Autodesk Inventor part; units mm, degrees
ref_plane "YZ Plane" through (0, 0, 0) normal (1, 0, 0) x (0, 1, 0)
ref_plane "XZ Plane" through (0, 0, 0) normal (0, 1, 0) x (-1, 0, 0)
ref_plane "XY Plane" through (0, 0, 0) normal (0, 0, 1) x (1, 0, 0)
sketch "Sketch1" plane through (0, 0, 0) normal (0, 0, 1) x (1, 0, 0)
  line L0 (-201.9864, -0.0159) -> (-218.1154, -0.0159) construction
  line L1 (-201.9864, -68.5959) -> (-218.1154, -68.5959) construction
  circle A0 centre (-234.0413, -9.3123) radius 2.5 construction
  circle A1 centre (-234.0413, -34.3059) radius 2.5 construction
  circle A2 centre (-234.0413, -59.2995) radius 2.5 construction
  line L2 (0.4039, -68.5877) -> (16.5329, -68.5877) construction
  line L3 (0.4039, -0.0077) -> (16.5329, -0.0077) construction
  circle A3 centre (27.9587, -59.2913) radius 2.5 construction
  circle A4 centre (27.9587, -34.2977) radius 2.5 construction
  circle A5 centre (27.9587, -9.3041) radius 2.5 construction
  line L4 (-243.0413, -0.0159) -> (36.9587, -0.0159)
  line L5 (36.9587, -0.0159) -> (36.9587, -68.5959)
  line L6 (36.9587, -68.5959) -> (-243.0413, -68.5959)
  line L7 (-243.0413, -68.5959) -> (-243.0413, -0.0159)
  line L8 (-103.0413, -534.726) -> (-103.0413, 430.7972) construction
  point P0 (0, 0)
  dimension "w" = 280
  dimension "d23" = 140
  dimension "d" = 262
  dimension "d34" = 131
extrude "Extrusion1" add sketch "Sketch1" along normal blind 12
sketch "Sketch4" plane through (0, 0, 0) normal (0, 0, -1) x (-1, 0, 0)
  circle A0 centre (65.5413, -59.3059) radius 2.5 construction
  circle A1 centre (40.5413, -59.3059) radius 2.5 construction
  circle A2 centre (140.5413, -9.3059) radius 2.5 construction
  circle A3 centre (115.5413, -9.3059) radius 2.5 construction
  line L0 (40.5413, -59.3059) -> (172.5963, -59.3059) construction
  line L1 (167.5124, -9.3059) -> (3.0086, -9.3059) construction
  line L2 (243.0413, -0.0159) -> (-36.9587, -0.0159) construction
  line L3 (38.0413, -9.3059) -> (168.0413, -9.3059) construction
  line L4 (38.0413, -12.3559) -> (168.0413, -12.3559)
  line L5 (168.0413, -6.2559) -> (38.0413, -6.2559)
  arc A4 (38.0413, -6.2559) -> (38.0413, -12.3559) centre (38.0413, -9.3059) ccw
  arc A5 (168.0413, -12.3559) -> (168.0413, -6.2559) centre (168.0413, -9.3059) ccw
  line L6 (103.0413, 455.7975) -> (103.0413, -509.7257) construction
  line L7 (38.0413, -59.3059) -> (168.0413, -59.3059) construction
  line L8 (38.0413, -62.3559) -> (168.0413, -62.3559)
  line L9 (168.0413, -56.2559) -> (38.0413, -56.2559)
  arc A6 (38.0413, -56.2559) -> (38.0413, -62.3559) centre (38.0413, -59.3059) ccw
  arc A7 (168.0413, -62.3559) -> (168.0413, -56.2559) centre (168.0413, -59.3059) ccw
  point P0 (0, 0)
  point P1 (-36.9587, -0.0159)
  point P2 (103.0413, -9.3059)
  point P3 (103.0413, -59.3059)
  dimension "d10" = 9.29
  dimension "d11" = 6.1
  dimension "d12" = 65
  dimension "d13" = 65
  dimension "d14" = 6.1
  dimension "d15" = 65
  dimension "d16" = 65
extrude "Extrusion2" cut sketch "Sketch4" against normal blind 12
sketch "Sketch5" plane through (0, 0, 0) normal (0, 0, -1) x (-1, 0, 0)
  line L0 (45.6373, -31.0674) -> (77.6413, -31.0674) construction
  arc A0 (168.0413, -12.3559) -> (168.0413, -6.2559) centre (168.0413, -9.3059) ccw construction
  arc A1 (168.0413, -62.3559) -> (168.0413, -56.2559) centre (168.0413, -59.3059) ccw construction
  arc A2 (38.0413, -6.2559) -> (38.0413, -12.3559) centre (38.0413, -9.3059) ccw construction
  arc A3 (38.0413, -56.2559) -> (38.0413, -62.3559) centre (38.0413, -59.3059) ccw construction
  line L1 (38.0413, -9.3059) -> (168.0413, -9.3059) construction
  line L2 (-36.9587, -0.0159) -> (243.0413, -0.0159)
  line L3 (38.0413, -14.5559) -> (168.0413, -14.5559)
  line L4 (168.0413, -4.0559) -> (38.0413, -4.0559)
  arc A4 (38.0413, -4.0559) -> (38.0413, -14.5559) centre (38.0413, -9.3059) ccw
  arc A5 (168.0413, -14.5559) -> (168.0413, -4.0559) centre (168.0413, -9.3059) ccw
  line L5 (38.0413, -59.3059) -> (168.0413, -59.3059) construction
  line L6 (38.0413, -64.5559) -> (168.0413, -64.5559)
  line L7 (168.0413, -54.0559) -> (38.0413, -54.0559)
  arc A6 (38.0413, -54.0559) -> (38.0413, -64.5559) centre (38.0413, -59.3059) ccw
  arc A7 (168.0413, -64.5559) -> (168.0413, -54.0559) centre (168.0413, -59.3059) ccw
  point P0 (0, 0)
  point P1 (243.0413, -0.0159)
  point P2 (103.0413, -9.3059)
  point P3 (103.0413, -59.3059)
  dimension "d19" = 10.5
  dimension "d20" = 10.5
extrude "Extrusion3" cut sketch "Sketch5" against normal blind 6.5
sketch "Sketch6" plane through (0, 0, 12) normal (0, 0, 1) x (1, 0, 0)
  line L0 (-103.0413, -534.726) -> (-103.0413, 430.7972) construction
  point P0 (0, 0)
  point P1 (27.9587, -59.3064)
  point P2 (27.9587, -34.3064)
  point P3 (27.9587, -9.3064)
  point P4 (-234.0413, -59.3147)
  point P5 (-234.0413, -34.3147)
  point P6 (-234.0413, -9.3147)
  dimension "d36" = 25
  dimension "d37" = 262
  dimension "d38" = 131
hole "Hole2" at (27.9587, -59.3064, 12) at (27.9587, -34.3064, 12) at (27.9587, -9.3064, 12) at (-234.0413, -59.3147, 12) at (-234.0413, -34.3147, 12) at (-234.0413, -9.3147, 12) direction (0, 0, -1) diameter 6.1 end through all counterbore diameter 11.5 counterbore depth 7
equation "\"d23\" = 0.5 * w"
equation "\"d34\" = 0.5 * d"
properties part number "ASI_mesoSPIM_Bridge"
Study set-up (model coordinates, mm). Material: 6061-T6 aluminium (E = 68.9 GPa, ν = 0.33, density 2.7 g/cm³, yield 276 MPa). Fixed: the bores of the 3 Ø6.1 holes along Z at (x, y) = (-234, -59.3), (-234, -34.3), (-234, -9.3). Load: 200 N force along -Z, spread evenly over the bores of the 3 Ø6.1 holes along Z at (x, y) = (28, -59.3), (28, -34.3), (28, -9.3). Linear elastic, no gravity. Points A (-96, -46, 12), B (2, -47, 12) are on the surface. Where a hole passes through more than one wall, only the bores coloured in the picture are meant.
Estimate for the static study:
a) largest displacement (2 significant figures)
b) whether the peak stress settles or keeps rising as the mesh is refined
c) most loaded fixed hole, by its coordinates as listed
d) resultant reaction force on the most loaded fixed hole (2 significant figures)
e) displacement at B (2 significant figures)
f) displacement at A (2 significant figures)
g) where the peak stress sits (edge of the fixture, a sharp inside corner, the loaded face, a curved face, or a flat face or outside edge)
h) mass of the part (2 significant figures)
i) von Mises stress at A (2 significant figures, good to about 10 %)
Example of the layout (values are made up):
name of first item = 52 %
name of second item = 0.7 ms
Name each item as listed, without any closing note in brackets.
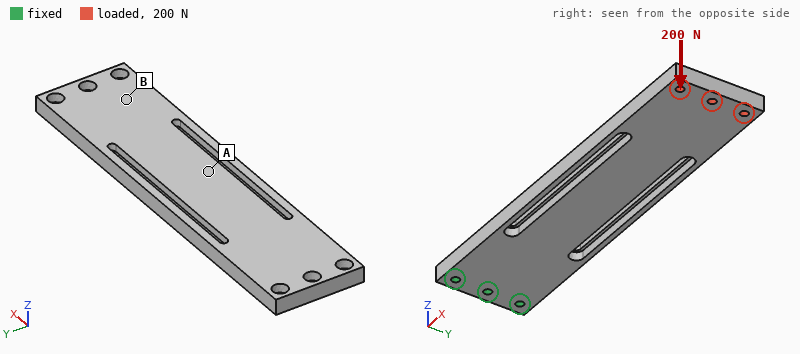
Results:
largest displacement = 2.6 mm
whether the peak stress settles or keeps rising as the mesh is refined = keeps rising
most loaded fixed hole, by its coordinates as listed = (-234, -34.3)
resultant reaction force on the most loaded fixed hole = 440 N
displacement at B = 2.1 mm
displacement at A = 0.91 mm
where the peak stress sits = edge of the fixture
mass of the part = 530 g
von Mises stress at A = 19 MPa
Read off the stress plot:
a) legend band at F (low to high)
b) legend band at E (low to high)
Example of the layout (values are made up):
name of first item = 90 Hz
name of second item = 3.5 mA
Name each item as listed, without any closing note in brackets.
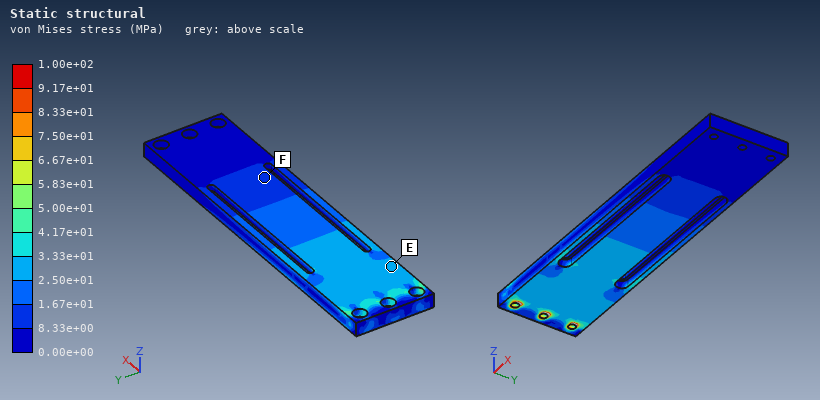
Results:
legend band at F = 8.33e+00 to 1.67e+01 MPa
legend band at E = 2.50e+01 to 3.33e+01 MPa
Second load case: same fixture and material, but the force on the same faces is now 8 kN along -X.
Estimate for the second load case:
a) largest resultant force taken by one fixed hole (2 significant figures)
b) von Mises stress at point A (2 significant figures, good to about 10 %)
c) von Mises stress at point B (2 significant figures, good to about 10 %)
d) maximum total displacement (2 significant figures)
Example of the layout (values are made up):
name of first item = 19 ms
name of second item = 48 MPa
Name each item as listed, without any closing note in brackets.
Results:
largest resultant force taken by one fixed hole = 2.8 kN
von Mises stress at point A = 10 MPa
von Mises stress at point B = 7.0 MPa
maximum total displacement = 1.8 mm
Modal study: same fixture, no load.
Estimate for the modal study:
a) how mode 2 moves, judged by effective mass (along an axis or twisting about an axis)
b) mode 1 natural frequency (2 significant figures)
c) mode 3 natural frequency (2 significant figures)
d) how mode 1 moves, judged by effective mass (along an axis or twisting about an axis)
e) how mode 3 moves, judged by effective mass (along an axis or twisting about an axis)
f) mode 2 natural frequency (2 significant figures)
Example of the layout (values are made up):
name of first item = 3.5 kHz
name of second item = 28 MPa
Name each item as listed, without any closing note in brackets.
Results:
how mode 2 moves, judged by effective mass = along Y
mode 1 natural frequency = 120 Hz
mode 3 natural frequency = 750 Hz
how mode 1 moves, judged by effective mass = along Z
how mode 3 moves, judged by effective mass = along Z
mode 2 natural frequency = 590 Hz
